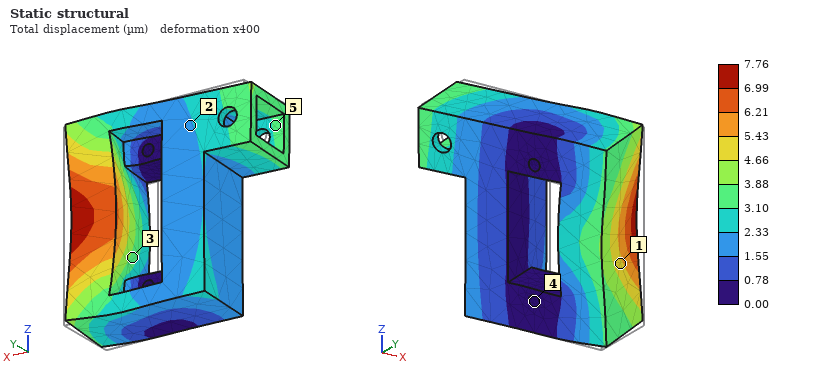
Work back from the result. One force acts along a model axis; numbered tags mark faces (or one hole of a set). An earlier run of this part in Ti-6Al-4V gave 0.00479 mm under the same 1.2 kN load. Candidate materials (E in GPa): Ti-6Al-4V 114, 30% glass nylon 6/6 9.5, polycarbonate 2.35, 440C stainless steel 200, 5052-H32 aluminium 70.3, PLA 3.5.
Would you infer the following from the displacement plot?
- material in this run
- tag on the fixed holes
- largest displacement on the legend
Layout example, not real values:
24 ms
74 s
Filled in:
5052-H32 aluminium
4
7.76 µm
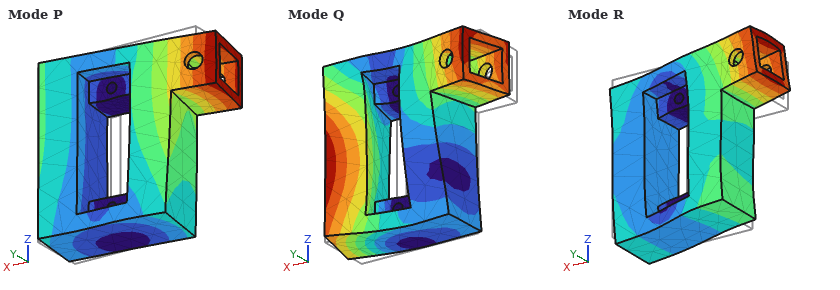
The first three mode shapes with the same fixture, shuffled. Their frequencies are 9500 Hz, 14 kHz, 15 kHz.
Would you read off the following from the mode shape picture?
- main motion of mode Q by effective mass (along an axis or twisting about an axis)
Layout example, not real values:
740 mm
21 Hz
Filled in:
along Y
